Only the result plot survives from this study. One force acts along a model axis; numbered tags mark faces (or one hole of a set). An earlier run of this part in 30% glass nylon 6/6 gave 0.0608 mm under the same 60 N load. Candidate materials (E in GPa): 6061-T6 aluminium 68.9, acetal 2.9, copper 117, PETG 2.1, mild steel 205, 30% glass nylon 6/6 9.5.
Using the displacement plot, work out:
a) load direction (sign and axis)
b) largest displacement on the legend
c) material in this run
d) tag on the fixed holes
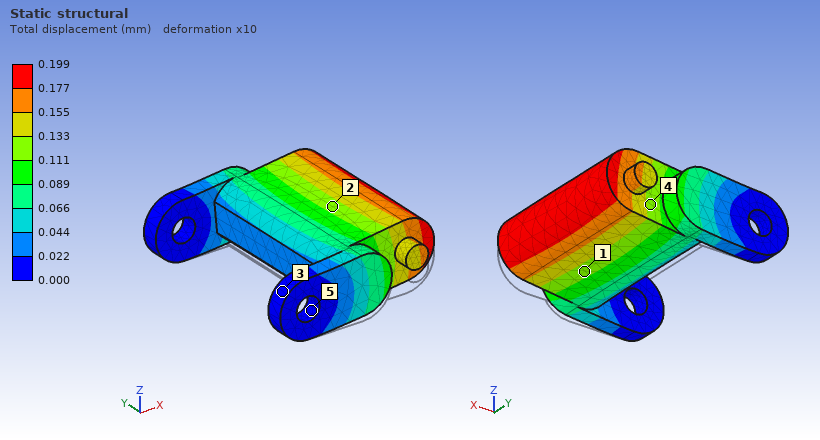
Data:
+Z
0.199 mm
acetal
5
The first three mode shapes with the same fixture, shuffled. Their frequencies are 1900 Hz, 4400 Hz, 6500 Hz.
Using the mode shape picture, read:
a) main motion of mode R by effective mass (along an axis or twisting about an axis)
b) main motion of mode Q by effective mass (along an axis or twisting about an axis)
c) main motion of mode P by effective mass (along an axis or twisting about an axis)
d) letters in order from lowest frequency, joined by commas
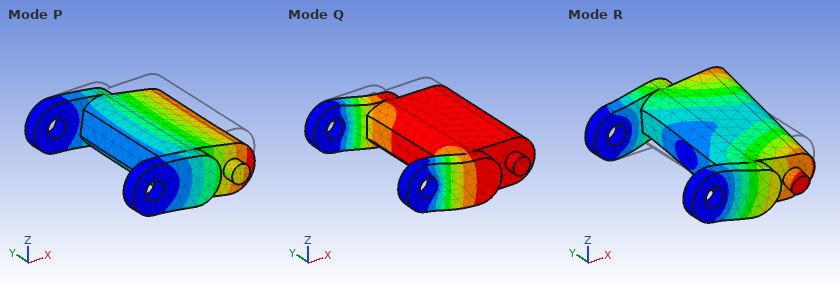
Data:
twisting about X
along Y
along Z
P, Q, R
